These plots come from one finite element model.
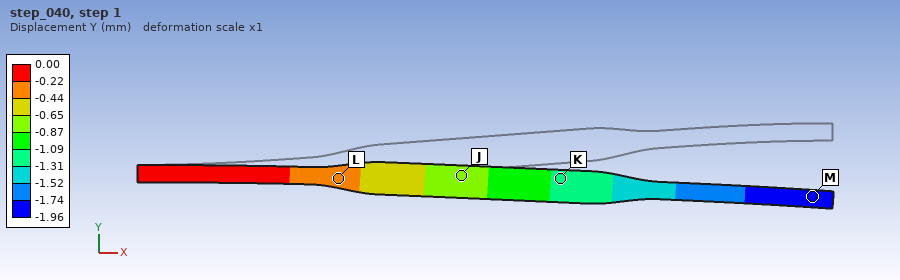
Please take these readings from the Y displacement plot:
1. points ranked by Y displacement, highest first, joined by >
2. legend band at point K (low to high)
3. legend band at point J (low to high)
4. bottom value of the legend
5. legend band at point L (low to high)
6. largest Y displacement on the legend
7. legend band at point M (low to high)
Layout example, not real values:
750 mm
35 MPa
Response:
L > J > K > M
-1.31 to -1.09 mm
-0.87 to -0.65 mm
-1.96 mm
-0.44 to -0.22 mm
0.00 mm
-1.96 to -1.74 mm
